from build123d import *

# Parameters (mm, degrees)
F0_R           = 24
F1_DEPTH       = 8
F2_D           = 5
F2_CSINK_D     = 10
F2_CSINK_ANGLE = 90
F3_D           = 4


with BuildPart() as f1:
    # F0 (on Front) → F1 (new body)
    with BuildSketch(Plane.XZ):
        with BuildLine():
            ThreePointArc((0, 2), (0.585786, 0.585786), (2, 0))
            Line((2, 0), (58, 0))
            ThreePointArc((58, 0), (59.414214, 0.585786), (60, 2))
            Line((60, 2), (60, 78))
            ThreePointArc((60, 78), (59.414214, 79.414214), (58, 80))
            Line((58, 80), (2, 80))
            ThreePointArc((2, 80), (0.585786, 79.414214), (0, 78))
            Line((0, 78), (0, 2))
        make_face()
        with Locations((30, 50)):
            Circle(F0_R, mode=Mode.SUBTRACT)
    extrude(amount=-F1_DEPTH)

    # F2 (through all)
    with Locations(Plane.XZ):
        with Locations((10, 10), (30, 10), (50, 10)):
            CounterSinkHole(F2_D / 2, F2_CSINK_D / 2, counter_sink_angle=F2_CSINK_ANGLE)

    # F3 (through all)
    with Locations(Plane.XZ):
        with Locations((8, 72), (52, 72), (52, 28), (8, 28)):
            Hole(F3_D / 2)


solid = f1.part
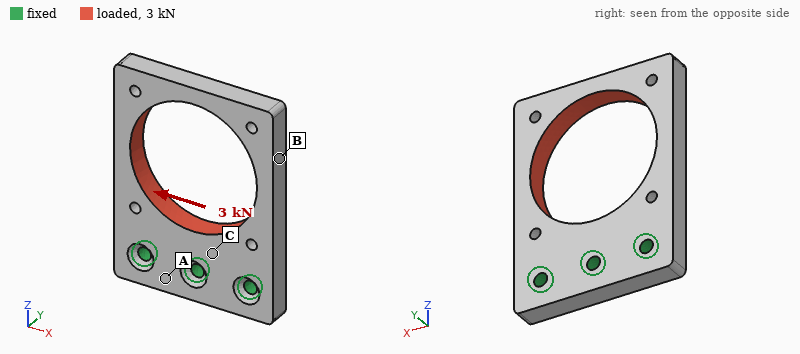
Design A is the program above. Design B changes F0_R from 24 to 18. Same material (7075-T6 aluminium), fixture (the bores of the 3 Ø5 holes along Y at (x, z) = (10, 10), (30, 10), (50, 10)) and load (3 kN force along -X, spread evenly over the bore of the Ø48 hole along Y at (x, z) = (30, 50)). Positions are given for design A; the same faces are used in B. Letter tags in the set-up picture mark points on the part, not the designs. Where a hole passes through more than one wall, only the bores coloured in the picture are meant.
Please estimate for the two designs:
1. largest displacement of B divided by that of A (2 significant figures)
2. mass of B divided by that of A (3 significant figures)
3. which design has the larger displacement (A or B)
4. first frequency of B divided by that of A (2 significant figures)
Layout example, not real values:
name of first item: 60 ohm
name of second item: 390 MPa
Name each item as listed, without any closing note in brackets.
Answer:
largest displacement of B divided by that of A: 0.33
mass of B divided by that of A: 1.28
which design has the larger displacement: A
first frequency of B divided by that of A: 1.1
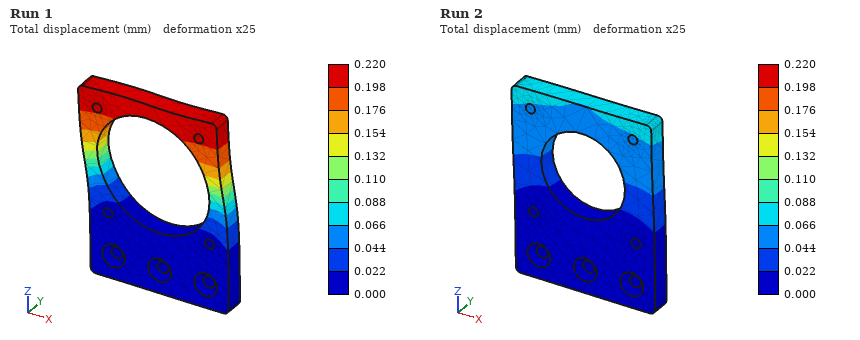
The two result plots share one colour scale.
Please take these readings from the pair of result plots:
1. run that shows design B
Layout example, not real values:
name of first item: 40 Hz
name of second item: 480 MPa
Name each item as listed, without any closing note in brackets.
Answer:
run that shows design B: Run 2
